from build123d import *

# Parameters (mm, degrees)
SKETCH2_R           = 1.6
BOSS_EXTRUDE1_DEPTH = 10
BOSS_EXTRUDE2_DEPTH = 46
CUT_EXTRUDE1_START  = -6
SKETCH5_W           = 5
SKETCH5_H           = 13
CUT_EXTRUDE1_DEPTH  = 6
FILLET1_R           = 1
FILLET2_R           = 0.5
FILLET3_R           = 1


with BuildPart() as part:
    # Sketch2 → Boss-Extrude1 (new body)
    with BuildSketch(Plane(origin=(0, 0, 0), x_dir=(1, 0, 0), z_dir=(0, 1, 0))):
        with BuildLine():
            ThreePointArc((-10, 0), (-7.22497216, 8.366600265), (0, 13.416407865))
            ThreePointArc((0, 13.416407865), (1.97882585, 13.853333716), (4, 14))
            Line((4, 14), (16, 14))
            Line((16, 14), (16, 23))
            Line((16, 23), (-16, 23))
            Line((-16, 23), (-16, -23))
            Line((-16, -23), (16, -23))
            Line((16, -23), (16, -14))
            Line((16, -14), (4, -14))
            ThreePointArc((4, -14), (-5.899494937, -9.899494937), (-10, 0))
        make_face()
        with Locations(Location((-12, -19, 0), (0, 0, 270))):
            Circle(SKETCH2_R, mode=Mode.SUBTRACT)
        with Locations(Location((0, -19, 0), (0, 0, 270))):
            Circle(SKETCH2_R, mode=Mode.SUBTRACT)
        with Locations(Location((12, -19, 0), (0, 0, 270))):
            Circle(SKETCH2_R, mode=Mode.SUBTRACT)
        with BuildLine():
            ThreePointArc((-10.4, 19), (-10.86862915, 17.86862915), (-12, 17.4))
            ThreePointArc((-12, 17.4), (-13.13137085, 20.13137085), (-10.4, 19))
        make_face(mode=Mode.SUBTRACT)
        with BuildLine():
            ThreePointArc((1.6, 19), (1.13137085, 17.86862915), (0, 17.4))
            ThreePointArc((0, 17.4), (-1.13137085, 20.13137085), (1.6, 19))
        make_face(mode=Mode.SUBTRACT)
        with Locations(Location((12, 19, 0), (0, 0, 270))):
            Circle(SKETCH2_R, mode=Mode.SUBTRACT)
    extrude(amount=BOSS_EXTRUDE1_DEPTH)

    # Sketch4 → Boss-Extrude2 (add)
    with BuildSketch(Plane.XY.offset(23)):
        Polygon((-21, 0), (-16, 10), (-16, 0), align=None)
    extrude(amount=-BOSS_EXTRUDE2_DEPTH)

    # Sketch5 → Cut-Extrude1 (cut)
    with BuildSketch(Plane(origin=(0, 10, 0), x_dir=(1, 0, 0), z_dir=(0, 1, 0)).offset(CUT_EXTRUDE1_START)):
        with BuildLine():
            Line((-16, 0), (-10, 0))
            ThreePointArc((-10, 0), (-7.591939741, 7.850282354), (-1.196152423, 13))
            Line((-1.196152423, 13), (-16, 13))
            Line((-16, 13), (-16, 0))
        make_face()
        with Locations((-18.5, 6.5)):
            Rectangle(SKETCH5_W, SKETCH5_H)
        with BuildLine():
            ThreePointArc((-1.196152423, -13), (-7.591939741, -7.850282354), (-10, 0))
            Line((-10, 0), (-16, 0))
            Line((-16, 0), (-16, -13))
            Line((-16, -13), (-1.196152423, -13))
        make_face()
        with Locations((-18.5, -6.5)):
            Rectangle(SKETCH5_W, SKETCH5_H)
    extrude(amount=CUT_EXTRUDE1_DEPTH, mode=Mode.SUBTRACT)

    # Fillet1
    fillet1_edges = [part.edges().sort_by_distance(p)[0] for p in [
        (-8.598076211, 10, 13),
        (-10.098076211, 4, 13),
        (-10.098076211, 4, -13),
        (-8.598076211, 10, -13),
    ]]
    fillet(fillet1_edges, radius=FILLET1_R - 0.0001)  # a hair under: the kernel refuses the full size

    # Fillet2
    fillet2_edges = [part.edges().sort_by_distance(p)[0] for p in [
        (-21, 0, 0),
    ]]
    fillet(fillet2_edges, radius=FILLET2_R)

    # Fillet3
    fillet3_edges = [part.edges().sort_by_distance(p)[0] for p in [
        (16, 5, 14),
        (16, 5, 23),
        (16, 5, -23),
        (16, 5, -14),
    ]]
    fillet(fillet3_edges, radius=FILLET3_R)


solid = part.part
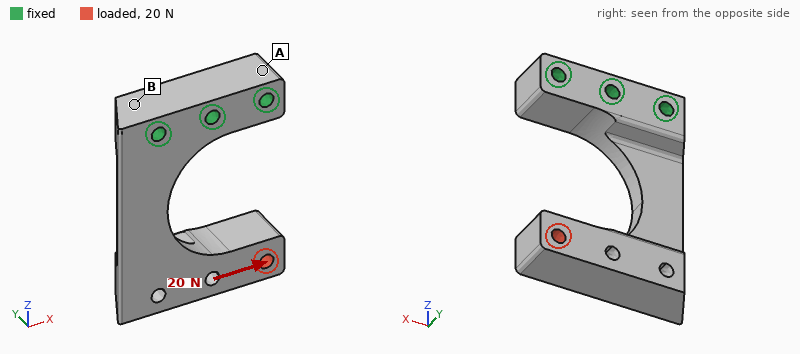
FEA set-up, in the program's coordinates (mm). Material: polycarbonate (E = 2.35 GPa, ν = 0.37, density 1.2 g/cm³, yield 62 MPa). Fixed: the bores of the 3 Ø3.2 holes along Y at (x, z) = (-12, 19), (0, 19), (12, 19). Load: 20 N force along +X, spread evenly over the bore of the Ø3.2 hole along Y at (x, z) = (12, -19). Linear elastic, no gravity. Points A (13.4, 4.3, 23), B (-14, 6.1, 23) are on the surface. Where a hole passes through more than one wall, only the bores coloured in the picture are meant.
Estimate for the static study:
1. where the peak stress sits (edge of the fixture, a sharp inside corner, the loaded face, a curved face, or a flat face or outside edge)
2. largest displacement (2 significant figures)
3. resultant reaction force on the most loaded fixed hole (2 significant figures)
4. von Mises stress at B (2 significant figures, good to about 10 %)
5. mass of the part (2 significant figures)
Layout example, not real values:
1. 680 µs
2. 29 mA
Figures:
1. a curved face
2. 0.59 mm
3. 54 N
4. 1.2 MPa
5. 8.9 g
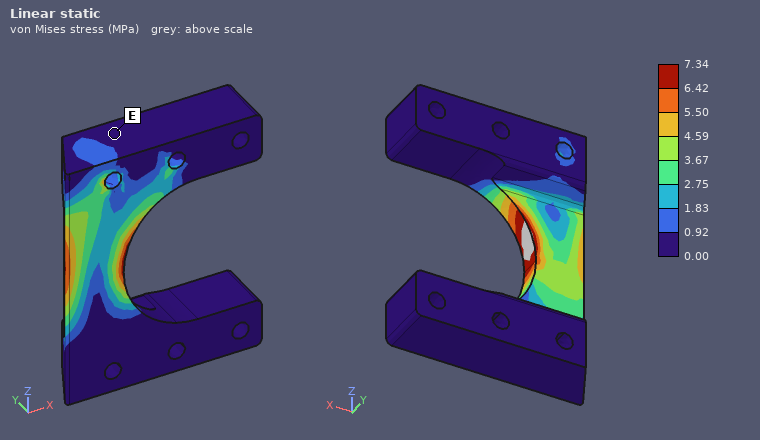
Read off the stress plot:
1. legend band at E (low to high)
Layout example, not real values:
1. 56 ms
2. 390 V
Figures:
1. 0.00 to 0.92 MPa
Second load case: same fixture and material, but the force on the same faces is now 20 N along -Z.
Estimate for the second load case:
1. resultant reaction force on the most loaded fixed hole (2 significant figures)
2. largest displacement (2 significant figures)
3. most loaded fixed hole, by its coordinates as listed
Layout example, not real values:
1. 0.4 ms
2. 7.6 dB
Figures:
1. 36 N
2. 0.68 mm
3. (0, 19)
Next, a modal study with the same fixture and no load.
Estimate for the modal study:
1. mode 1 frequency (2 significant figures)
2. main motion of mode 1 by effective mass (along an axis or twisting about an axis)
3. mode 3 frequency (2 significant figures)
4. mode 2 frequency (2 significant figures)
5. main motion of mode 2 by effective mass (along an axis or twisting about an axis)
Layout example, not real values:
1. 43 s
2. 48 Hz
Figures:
1. 250 Hz
2. along Y
3. 730 Hz
4. 570 Hz
5. along X
